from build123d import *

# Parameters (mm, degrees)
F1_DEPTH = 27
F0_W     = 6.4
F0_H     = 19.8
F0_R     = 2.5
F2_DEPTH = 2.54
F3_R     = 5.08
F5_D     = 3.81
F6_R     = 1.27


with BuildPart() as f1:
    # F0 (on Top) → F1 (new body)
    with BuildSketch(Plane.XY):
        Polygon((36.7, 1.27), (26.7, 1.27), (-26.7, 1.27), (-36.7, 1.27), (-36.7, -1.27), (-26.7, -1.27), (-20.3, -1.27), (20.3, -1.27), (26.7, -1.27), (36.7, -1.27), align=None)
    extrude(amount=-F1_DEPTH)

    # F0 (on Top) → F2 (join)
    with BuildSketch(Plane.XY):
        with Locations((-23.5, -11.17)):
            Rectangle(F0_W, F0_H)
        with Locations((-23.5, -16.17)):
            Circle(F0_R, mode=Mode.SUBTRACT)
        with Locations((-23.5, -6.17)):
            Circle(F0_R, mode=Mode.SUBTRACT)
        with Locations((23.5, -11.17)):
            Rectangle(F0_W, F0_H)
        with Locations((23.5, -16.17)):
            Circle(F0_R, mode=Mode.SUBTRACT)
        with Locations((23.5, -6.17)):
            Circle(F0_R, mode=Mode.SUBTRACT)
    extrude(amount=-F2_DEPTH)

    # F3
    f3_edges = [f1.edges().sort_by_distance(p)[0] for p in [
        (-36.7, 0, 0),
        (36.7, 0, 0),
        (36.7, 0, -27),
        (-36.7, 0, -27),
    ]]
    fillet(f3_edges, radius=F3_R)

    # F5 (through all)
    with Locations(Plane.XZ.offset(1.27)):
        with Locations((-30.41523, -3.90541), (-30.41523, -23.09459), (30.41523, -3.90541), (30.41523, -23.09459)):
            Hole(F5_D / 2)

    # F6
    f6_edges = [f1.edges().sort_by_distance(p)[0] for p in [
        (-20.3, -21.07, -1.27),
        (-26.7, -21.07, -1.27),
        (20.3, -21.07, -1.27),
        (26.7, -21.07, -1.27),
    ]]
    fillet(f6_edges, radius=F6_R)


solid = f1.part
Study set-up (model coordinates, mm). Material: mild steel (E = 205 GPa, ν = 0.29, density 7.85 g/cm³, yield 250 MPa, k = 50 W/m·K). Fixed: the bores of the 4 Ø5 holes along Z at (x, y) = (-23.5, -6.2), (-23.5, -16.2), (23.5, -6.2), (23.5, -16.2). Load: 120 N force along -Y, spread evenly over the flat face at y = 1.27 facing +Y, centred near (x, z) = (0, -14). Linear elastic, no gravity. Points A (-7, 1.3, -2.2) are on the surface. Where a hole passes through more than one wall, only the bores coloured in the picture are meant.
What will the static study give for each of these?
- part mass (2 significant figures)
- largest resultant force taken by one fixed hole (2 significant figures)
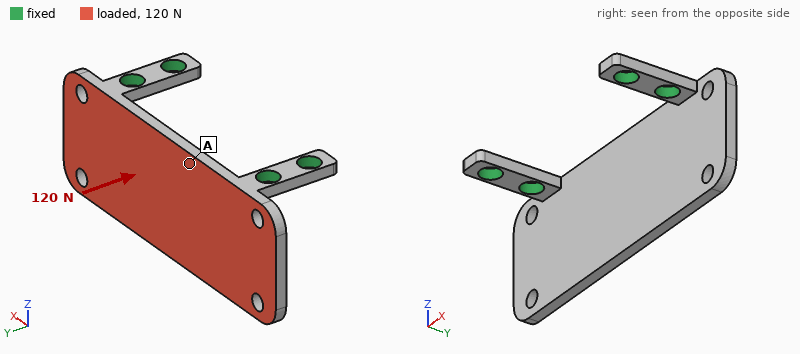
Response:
42 g
62 N
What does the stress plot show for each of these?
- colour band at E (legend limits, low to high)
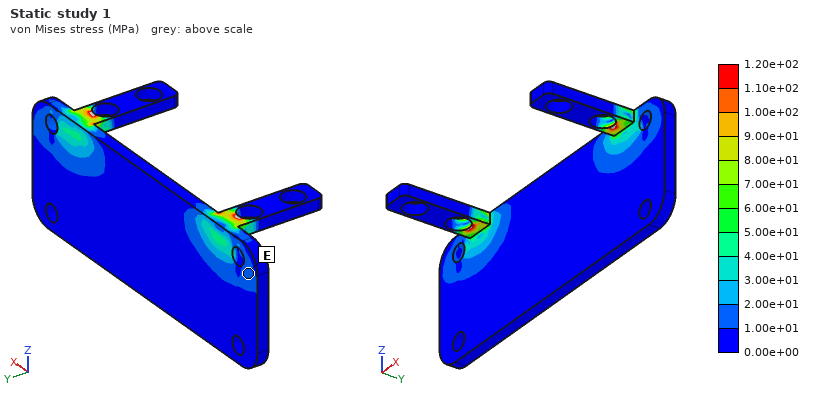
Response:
1.00e+01 to 2.00e+01 MPa
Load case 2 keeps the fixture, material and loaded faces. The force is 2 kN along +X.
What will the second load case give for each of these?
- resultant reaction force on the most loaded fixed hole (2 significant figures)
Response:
1.1 kN
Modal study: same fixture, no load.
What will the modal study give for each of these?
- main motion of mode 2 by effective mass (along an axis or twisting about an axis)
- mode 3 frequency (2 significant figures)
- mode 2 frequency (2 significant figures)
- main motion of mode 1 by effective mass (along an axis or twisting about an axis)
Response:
twisting about Z
4200 Hz
2800 Hz
along Y
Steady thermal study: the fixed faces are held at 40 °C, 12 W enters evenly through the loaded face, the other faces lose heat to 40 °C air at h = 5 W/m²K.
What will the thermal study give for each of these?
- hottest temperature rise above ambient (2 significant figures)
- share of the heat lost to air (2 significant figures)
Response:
58 K
5.1 %
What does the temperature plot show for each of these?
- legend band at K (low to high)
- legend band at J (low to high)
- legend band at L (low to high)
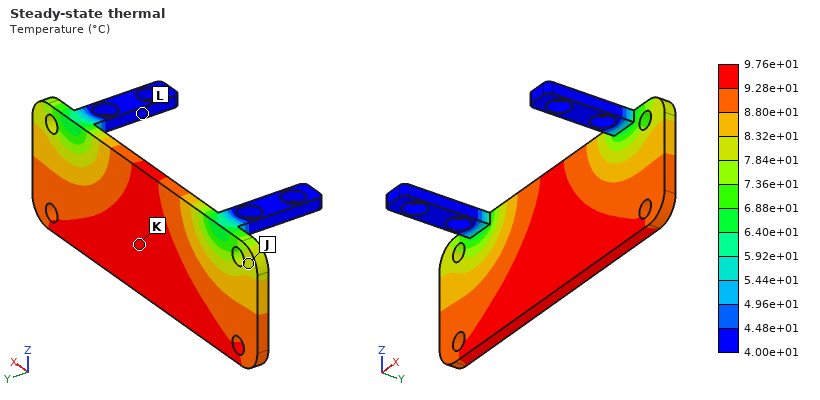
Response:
9.28e+01 to 9.76e+01 °C
7.84e+01 to 8.32e+01 °C
4.00e+01 to 4.48e+01 °C
